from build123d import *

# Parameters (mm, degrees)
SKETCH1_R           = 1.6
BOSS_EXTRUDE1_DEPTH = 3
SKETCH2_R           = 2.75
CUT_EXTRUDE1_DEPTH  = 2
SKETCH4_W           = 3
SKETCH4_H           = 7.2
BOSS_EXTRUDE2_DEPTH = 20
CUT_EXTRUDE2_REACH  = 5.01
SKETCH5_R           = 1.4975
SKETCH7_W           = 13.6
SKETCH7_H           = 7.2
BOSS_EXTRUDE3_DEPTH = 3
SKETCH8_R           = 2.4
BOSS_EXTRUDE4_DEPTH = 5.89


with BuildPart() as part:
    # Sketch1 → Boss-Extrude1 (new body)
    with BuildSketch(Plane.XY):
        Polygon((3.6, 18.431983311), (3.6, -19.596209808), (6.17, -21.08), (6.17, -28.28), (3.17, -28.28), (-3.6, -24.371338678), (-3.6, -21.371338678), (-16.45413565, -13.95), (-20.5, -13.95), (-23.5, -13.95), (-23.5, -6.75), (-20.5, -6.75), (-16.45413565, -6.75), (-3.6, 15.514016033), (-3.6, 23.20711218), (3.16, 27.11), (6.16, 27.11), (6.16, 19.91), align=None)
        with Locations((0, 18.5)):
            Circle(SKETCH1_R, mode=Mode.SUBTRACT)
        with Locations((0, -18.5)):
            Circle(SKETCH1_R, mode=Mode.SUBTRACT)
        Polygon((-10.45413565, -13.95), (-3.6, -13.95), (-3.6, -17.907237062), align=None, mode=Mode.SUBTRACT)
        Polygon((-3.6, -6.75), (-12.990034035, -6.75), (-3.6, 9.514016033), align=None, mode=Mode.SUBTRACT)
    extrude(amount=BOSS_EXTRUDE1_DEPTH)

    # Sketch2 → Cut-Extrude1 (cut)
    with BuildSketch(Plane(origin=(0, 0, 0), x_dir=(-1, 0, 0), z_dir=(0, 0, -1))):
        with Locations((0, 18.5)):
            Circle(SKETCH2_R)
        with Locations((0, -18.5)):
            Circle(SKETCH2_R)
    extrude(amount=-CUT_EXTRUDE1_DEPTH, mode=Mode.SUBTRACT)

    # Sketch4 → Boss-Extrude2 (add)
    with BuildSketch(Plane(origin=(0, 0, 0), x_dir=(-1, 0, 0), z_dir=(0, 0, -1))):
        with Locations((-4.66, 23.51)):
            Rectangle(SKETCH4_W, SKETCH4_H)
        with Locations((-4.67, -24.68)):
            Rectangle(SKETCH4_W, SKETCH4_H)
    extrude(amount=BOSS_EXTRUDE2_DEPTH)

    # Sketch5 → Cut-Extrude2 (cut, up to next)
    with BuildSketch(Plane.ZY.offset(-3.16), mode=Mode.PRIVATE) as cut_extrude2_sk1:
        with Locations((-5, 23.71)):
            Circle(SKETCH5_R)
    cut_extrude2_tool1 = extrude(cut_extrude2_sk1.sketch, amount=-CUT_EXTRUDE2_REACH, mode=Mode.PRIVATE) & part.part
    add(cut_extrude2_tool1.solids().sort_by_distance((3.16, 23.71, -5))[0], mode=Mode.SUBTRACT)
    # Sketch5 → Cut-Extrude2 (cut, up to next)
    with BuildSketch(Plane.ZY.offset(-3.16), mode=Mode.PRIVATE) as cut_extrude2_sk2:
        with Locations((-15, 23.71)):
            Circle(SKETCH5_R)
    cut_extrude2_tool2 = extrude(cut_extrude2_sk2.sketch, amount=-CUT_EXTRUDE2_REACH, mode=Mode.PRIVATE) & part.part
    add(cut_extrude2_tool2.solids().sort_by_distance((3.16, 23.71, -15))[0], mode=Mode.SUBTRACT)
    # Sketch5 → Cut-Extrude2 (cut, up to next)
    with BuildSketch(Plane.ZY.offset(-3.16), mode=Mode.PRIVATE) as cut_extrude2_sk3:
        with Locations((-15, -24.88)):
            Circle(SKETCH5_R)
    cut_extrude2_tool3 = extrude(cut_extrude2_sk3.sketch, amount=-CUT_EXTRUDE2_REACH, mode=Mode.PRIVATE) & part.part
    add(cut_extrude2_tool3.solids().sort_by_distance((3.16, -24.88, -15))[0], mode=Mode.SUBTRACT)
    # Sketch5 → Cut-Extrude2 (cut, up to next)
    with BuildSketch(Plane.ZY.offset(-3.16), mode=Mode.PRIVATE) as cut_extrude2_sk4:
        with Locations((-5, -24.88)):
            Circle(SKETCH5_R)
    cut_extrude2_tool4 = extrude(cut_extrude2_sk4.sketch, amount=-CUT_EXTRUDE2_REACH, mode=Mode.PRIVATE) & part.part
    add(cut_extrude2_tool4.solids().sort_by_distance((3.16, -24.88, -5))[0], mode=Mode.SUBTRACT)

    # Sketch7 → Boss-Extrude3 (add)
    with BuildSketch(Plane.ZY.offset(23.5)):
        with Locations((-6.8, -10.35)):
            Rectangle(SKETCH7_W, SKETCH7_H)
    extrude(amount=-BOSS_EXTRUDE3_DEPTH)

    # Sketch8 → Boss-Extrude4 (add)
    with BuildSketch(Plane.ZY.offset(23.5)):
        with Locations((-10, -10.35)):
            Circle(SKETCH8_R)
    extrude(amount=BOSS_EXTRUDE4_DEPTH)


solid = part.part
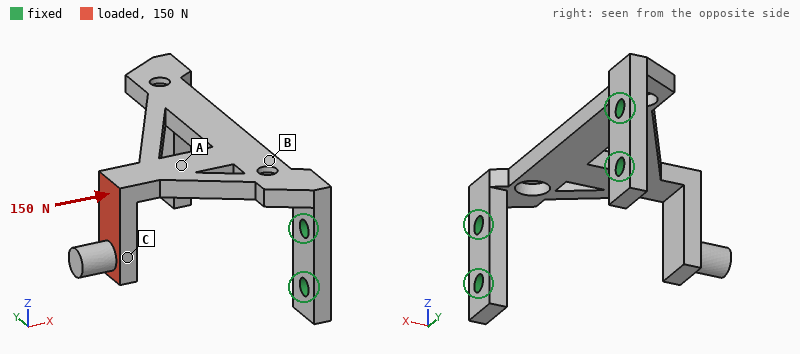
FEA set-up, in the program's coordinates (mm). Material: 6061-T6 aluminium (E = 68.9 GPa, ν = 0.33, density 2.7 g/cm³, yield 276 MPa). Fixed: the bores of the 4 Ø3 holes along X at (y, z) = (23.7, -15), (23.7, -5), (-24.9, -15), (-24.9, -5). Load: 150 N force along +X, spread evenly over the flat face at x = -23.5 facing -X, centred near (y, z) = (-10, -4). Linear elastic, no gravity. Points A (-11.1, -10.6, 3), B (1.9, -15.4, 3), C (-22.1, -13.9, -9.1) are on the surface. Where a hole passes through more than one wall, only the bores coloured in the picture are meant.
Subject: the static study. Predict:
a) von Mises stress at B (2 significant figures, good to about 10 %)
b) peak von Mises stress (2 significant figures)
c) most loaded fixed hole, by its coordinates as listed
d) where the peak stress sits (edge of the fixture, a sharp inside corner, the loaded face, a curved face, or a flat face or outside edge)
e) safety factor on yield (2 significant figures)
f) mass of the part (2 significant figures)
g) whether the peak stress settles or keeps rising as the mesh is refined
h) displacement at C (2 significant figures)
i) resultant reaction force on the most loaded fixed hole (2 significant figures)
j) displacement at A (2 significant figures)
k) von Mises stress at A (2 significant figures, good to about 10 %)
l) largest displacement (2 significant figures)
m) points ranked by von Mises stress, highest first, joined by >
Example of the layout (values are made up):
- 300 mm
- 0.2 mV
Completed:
- 37 MPa
- 180 MPa
- (-24.9, -5)
- a curved face
- 1.6
- 8.2 g
- settles
- 0.38 mm
- 120 N
- 0.12 mm
- 55 MPa
- 0.56 mm
- A > B > C
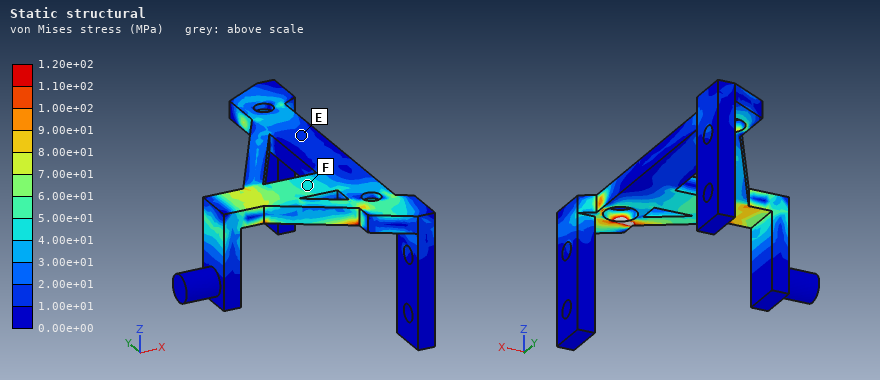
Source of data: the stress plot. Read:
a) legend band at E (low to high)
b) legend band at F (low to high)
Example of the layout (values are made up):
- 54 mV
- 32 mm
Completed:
- 1.00e+01 to 2.00e+01 MPa
- 4.00e+01 to 5.00e+01 MPa
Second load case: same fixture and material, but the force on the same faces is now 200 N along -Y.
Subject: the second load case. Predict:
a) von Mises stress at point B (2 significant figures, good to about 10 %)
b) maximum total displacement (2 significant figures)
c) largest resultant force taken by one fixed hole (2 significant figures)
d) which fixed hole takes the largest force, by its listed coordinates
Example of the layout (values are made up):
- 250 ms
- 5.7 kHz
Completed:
- 31 MPa
- 0.26 mm
- 200 N
- (23.7, -5)
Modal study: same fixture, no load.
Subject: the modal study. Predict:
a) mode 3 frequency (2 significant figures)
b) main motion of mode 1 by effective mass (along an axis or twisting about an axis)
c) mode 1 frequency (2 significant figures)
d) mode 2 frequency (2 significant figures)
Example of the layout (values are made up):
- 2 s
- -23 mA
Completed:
- 4400 Hz
- along Z
- 1200 Hz
- 3700 Hz
